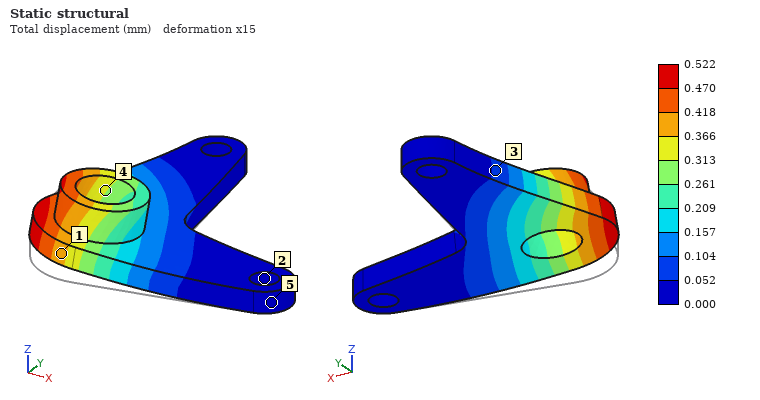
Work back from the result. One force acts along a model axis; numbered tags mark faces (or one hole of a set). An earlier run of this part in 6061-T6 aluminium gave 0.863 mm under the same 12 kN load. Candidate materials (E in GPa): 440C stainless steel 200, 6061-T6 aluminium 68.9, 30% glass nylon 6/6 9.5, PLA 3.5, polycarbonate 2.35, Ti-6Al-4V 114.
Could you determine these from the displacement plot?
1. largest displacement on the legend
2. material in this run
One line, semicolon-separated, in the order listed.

0.522 mm; Ti-6Al-4V
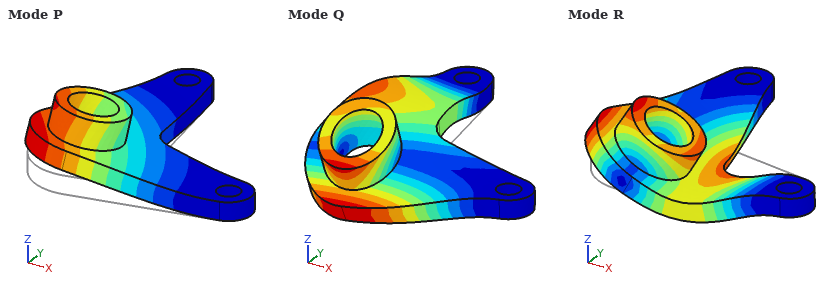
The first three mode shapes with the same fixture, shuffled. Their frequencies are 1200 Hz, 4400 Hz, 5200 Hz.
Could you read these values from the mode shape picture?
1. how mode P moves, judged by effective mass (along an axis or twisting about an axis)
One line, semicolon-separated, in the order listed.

along Z
